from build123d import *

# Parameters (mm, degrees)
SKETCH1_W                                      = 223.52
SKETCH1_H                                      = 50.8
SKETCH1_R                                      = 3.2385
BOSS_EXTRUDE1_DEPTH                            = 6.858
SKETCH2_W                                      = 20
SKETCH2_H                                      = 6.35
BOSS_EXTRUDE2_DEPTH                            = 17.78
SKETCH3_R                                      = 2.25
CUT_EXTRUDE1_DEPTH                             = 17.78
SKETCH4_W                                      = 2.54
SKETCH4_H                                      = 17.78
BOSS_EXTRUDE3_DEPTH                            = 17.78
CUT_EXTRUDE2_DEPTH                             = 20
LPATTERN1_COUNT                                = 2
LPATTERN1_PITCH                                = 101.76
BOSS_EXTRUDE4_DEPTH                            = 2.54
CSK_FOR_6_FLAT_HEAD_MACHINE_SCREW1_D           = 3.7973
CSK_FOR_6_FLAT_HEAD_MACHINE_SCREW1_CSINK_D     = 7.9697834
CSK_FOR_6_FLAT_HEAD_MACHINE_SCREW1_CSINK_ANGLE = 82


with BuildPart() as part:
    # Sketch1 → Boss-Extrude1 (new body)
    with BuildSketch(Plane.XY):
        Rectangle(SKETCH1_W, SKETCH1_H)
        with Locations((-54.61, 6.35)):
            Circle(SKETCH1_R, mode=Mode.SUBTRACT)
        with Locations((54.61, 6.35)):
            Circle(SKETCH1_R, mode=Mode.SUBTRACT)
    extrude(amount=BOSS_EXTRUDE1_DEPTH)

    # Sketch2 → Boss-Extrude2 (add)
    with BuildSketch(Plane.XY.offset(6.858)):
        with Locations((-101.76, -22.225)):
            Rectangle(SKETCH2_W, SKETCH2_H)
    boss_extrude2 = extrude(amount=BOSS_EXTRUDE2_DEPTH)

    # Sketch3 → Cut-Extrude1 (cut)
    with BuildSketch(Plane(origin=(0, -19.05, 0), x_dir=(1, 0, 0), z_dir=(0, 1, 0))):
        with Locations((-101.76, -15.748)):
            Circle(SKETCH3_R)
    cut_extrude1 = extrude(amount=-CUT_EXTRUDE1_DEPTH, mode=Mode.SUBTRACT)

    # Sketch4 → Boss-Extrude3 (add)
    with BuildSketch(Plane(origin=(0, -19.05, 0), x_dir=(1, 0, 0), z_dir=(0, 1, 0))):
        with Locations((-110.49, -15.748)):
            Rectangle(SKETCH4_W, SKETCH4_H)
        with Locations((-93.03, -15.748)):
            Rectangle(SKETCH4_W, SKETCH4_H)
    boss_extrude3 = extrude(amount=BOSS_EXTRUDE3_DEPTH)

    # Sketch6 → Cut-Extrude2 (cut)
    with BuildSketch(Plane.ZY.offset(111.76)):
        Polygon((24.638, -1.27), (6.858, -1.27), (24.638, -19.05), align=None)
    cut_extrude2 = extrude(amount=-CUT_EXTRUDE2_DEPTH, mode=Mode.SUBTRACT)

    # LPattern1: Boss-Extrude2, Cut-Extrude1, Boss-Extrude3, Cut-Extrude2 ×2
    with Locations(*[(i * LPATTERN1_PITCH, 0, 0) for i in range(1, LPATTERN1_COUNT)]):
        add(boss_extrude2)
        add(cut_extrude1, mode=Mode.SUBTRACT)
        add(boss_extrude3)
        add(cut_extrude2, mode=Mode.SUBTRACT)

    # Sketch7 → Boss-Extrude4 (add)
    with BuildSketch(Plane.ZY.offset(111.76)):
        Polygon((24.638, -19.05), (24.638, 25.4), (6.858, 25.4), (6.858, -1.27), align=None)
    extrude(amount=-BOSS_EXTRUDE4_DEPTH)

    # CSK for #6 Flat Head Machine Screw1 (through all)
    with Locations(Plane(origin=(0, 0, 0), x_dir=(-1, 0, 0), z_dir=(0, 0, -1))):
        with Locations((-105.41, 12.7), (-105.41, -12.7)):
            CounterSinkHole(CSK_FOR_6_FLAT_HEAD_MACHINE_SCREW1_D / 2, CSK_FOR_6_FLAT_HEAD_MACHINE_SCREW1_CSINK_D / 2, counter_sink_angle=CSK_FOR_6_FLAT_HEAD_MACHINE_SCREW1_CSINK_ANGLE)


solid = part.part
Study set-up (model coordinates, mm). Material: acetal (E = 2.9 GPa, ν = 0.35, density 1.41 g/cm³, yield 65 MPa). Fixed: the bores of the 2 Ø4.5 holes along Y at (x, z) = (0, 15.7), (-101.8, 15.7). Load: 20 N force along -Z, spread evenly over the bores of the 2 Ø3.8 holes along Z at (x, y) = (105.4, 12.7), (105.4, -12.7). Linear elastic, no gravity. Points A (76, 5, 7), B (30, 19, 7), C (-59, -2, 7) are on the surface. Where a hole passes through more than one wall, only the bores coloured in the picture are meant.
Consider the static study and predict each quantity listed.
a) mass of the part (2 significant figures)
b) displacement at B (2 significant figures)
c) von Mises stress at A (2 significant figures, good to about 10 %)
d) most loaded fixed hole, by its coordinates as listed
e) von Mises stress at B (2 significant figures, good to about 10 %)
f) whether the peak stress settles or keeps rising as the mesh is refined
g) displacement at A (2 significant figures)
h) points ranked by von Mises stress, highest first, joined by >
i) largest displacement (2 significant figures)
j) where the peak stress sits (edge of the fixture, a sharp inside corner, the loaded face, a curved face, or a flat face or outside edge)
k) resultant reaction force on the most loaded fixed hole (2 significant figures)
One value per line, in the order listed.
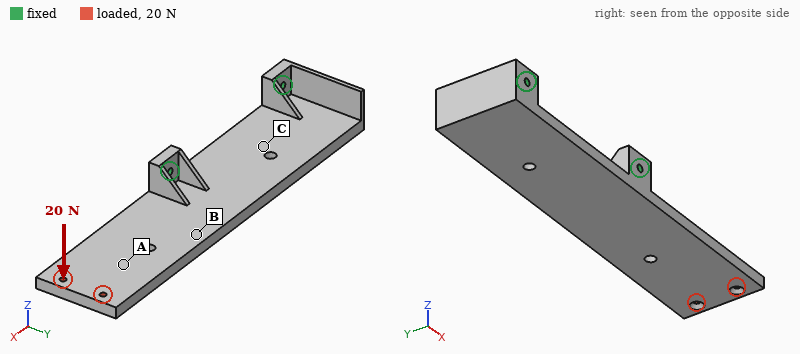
120 g
0.42 mm
1.5 MPa
(0, 15.7)
3.4 MPa
keeps rising
1.5 mm
B > A > C
2.6 mm
edge of the fixture
54 N
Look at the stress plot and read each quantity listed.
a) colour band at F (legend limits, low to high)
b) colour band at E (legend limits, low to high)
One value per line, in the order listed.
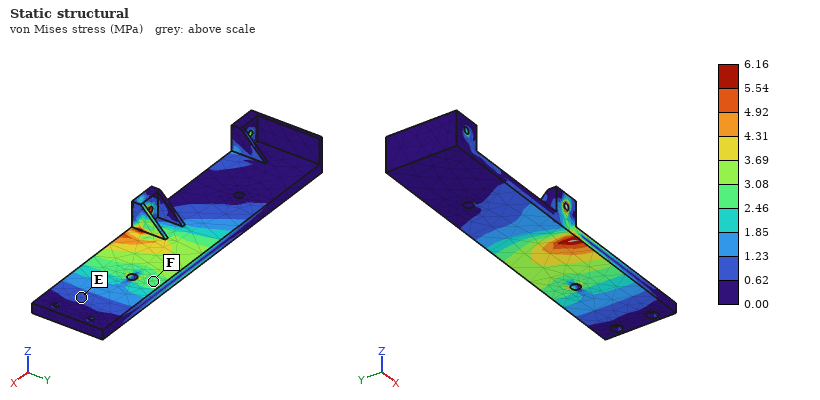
2.46 to 3.08 MPa
0.62 to 1.23 MPa
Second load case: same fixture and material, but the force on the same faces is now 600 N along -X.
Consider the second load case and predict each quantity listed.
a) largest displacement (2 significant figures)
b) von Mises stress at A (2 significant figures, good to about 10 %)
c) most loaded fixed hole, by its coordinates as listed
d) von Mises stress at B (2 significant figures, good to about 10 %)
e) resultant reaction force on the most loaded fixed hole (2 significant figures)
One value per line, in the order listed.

1.0 mm
3.5 MPa
(0, 15.7)
3.3 MPa
370 N
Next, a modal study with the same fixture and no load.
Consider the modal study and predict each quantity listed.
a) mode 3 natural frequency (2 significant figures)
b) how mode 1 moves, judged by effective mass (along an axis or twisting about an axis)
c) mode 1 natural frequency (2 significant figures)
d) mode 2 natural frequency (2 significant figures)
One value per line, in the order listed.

470 Hz
along Z
110 Hz
340 Hz
